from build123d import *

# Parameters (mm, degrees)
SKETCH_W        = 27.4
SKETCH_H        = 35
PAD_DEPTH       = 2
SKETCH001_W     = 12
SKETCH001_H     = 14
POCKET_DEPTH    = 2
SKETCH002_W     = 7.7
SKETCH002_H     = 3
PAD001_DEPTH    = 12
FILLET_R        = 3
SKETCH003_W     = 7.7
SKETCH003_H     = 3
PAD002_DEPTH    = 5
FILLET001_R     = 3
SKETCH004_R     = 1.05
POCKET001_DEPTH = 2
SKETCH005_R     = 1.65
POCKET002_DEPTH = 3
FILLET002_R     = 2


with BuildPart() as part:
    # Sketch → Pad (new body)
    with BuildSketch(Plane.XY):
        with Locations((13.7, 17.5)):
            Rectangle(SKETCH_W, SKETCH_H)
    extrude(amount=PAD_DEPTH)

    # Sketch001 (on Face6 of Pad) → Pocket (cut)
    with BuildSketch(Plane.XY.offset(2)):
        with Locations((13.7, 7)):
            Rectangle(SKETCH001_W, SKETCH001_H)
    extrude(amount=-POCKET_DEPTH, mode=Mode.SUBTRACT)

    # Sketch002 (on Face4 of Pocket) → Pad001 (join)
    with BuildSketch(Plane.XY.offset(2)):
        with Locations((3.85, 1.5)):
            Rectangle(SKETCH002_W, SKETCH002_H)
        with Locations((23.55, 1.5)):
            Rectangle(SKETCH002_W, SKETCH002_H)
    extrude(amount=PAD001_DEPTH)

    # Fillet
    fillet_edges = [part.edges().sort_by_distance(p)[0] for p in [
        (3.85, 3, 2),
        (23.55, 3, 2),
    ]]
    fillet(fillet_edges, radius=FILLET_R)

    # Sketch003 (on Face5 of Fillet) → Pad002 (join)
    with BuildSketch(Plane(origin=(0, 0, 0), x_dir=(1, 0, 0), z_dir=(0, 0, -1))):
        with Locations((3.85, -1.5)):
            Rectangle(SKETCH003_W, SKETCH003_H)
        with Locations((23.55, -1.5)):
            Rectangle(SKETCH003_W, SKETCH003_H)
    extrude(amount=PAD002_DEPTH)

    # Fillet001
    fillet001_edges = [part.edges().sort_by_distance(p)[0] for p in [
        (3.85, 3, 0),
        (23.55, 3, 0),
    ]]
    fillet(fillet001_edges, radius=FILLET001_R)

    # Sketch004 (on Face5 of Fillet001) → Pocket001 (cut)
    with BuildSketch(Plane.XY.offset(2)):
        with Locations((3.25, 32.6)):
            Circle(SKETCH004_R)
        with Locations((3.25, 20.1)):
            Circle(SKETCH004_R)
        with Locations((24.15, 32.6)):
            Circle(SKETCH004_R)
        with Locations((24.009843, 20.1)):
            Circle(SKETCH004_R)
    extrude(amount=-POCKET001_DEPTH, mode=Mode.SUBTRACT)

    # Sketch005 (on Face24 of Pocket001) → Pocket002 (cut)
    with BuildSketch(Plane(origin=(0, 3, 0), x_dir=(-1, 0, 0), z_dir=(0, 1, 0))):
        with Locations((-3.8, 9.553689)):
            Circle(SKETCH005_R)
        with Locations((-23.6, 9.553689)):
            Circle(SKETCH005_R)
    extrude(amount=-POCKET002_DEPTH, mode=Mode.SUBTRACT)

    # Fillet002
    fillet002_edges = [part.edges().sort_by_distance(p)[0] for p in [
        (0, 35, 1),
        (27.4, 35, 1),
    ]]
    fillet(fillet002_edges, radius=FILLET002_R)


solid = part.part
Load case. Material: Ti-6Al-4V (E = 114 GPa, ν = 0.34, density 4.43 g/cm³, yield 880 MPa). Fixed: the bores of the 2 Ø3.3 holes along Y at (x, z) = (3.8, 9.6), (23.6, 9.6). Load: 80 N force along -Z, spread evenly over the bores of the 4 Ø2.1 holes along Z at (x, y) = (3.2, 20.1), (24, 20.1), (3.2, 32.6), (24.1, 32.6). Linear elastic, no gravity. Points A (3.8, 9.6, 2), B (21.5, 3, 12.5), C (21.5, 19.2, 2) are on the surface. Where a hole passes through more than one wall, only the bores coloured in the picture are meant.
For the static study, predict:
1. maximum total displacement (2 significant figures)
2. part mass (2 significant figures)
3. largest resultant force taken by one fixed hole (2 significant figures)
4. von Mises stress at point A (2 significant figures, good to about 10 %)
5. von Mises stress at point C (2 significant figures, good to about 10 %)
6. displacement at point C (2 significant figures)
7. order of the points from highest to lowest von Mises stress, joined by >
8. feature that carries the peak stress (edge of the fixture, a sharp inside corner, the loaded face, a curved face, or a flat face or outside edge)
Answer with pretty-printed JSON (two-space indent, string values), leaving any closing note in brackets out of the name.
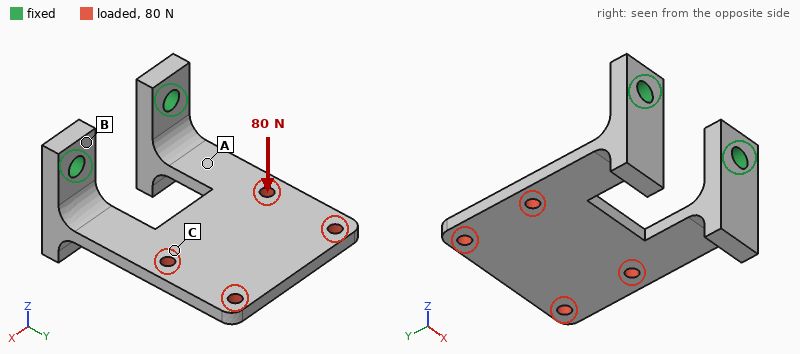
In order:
{
  "maximum total displacement": "0.47 mm",
  "part mass": "10 g",
  "largest resultant force taken by one fixed hole": "40 N",
  "von Mises stress at point A": "130 MPa",
  "von Mises stress at point C": "39 MPa",
  "displacement at point C": "0.18 mm",
  "order of the points from highest to lowest von Mises stress, joined by >": "A > C > B",
  "feature that carries the peak stress": "a curved face"
}
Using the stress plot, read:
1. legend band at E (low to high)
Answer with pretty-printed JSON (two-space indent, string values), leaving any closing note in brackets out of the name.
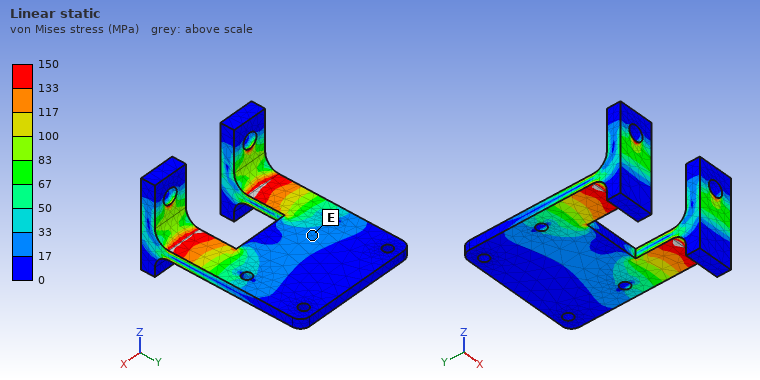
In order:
{
  "legend band at E": "17 to 33 MPa"
}
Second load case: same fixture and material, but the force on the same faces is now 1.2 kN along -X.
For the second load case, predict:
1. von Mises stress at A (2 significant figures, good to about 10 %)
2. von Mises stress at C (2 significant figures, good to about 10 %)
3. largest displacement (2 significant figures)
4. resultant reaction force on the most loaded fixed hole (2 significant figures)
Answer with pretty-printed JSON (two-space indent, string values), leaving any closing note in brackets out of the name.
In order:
{
  "von Mises stress at A": "280 MPa",
  "von Mises stress at C": "95 MPa",
  "largest displacement": "0.38 mm",
  "resultant reaction force on the most loaded fixed hole": "1.2 kN"
}
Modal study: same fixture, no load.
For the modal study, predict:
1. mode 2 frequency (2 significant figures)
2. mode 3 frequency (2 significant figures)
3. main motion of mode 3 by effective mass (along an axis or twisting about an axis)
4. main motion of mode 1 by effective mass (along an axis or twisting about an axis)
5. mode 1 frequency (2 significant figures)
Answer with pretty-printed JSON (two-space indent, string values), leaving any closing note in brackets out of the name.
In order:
{
  "mode 2 frequency": "3700 Hz",
  "mode 3 frequency": "5100 Hz",
  "main motion of mode 3 by effective mass": "along X",
  "main motion of mode 1 by effective mass": "along Z",
  "mode 1 frequency": "1200 Hz"
}
